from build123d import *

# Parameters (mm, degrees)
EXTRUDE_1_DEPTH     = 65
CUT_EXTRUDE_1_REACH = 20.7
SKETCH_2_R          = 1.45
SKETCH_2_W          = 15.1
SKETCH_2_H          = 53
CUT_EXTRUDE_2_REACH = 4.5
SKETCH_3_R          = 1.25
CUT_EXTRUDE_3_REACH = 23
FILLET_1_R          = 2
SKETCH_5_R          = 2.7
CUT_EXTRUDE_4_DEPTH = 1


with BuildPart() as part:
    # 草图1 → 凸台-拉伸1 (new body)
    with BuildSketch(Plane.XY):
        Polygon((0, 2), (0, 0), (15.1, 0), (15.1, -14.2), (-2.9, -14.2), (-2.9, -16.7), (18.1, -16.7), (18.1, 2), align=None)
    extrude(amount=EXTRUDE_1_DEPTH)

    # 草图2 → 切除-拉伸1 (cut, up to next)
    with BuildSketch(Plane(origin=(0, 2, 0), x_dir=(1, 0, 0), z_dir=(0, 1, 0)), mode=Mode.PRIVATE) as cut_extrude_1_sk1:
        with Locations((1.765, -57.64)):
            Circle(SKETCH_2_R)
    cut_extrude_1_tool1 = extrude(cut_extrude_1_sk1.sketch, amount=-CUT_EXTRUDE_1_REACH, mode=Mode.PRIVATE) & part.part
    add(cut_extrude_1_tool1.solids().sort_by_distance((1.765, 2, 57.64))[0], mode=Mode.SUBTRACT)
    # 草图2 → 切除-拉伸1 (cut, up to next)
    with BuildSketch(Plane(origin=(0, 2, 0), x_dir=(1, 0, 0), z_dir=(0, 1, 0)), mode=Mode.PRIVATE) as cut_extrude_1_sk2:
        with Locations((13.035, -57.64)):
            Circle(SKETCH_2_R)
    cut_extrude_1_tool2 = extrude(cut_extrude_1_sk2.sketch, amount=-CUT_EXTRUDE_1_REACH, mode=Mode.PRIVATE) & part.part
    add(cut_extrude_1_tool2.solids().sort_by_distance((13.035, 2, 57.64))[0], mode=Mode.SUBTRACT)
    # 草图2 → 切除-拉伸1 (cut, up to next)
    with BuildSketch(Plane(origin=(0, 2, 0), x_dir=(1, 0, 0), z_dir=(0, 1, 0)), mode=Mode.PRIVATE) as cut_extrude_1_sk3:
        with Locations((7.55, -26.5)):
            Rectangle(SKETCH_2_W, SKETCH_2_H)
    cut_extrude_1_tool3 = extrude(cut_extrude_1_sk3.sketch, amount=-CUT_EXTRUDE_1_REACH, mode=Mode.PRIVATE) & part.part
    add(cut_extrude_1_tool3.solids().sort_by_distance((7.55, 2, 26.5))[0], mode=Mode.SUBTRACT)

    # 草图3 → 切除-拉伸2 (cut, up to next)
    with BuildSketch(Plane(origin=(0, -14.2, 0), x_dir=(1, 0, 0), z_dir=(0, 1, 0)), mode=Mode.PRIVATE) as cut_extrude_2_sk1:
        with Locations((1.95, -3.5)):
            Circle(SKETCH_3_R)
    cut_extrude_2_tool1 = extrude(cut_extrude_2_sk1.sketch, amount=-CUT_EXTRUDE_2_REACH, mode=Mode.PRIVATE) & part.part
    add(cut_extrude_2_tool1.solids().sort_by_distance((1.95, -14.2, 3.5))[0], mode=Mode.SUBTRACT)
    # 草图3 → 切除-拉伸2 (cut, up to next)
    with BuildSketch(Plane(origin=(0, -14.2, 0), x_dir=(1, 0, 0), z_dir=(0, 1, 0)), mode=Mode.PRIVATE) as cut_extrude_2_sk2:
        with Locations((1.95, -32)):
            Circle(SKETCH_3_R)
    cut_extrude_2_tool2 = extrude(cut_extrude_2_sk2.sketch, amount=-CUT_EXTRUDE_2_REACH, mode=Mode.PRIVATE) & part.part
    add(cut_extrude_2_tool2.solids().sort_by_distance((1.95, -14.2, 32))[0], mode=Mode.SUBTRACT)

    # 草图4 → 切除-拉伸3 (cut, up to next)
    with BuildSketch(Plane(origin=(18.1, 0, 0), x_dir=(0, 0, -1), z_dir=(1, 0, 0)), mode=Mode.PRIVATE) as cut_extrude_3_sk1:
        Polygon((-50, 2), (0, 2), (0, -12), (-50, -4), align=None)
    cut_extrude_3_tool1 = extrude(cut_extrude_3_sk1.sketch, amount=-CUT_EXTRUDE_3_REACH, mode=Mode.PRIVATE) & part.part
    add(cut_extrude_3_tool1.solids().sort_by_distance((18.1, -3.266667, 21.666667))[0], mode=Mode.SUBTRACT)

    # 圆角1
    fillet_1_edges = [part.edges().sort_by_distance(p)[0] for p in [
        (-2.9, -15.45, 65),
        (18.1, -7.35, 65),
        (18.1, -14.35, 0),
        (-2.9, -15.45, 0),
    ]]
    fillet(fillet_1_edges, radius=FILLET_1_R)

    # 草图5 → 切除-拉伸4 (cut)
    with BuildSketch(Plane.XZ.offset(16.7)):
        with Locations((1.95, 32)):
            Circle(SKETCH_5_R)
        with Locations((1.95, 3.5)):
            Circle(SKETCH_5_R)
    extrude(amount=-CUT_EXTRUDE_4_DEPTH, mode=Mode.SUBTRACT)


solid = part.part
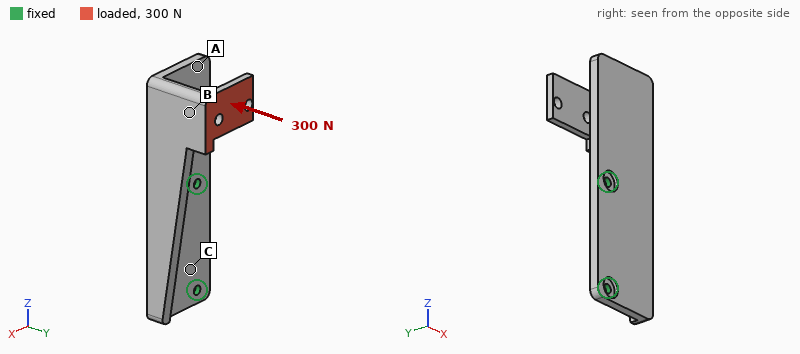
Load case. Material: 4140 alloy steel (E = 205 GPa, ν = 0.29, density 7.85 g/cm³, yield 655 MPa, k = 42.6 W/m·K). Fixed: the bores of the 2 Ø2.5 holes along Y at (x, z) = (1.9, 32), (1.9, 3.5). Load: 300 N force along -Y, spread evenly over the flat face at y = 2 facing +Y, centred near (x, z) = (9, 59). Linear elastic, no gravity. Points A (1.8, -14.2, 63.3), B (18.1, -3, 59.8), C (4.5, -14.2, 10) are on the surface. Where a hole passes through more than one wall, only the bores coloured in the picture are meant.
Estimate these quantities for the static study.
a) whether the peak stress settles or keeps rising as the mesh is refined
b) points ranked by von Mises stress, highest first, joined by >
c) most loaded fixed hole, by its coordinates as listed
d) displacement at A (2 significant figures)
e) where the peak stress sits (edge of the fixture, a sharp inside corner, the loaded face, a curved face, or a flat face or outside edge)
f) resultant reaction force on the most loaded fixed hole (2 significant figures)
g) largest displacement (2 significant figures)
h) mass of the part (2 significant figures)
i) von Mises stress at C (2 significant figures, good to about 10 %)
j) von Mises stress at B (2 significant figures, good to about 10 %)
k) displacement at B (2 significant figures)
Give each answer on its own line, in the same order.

keeps rising
B > C > A
(1.9, 32)
0.17 mm
edge of the fixture
570 N
0.35 mm
42 g
55 MPa
88 MPa
0.22 mm
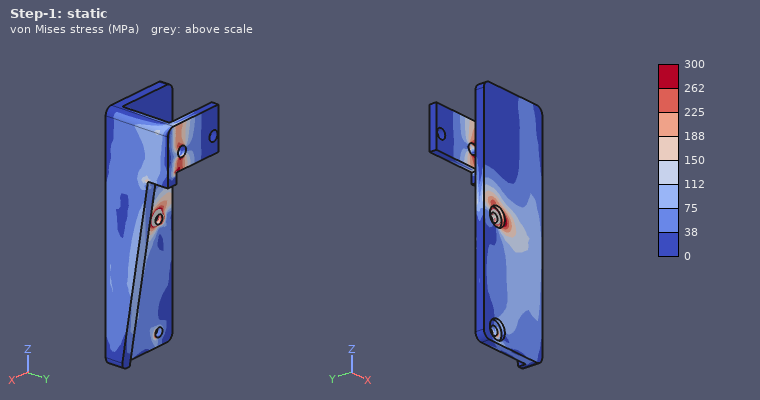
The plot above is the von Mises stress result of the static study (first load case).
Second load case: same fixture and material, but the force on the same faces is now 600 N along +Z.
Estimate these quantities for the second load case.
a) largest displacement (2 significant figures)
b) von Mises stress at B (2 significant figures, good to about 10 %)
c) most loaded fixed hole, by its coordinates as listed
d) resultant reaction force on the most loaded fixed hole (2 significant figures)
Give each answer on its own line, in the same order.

0.33 mm
150 MPa
(1.9, 32)
730 N
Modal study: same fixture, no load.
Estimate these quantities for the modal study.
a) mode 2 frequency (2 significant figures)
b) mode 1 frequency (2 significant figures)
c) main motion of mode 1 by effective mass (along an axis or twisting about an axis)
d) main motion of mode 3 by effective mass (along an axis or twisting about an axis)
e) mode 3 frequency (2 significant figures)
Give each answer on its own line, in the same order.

2200 Hz
1400 Hz
along Y
along Y
3800 Hz
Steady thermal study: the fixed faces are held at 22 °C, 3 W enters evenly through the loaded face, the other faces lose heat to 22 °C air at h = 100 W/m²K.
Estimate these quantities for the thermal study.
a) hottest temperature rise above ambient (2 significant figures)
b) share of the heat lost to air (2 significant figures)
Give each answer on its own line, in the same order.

33 K
85 %
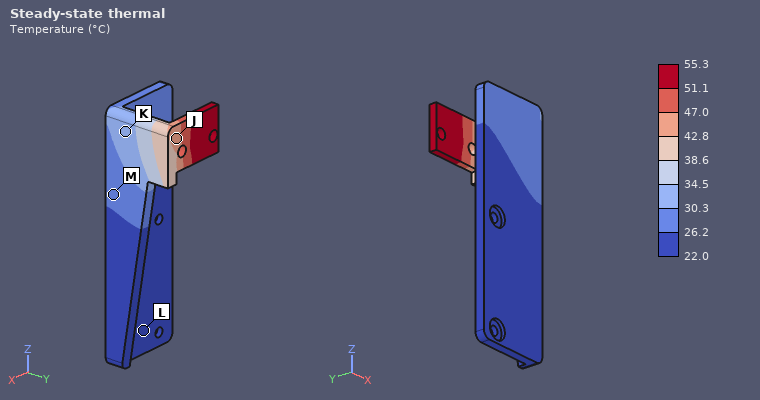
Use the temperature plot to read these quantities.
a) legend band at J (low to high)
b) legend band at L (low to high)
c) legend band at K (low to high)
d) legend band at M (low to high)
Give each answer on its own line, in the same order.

42.8 to 47.0 °C
22.0 to 26.2 °C
30.3 to 34.5 °C
26.2 to 30.3 °C
